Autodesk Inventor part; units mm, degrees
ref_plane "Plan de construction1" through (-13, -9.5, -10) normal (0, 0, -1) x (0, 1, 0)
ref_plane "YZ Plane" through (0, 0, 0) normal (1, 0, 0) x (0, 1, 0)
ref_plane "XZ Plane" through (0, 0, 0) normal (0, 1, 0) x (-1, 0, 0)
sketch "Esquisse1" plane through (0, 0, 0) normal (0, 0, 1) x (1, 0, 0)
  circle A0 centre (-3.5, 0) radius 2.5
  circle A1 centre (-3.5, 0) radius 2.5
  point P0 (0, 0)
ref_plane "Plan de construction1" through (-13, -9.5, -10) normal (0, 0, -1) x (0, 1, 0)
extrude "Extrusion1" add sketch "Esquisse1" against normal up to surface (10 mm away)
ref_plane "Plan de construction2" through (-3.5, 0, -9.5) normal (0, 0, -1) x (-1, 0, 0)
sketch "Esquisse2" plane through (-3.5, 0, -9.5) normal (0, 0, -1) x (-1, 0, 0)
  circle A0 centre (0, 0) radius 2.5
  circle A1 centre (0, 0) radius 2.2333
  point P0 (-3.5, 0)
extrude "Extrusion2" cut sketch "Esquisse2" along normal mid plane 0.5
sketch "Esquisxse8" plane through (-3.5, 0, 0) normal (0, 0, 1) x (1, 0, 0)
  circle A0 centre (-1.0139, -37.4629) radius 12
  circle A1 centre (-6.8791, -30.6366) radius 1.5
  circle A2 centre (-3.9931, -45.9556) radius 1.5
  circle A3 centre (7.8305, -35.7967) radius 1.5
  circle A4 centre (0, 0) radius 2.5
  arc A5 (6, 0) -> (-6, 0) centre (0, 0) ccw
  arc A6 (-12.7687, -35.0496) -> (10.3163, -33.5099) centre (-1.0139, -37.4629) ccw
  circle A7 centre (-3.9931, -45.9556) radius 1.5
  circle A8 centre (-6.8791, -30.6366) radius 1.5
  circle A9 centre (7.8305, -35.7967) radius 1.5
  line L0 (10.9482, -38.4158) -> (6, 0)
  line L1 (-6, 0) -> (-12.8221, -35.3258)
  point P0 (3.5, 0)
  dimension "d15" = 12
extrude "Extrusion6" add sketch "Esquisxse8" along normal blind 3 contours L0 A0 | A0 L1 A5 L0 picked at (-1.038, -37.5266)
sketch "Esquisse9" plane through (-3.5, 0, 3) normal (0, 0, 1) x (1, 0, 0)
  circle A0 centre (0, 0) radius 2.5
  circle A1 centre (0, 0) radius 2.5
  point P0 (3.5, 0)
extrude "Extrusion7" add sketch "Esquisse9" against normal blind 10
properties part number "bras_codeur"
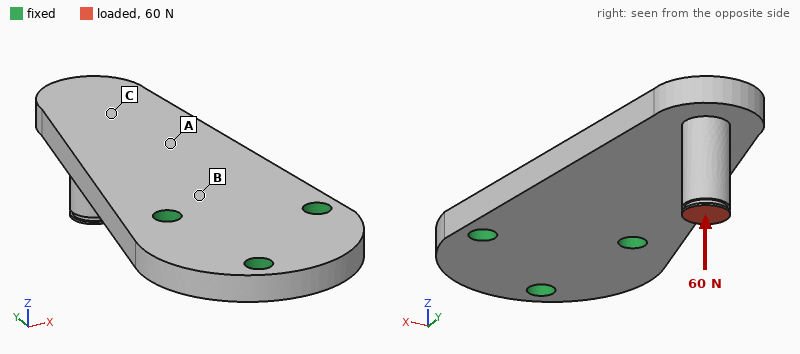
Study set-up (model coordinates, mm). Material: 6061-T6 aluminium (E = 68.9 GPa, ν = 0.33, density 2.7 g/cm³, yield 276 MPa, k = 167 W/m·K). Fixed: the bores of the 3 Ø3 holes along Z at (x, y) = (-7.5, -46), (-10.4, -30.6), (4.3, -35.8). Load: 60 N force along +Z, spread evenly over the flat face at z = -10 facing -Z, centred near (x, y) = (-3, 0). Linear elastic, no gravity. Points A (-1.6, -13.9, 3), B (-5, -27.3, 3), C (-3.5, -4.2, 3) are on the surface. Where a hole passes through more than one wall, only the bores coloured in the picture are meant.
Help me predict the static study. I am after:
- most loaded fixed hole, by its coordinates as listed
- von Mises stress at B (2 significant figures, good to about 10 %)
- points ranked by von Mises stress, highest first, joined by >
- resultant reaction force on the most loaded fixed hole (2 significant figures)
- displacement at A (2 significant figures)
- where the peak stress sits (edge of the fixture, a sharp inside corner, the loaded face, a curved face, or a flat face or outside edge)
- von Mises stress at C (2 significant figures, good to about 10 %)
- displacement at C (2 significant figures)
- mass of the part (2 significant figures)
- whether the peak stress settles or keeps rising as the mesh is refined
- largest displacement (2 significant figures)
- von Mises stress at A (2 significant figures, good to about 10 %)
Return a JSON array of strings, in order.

["(-10.4, -30.6)", "47 MPa", "B > A > C", "89 N", "0.084 mm", "edge of the fixture", "14 MPa", "0.17 mm", "8.1 g", "keeps rising", "0.28 mm", "33 MPa"]
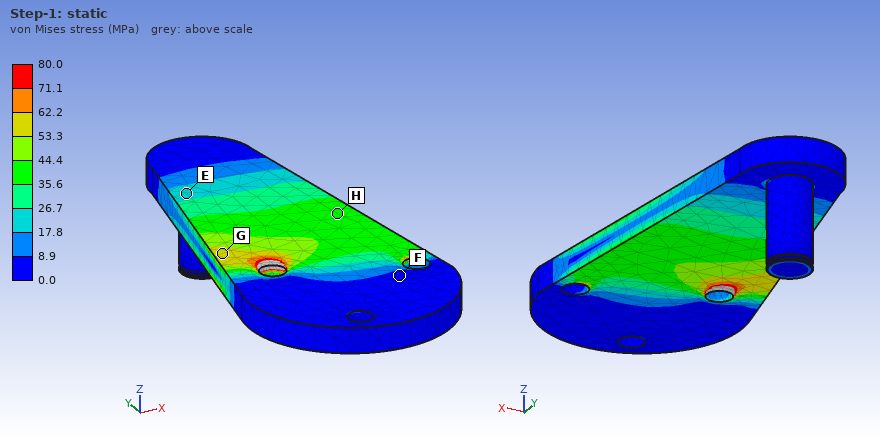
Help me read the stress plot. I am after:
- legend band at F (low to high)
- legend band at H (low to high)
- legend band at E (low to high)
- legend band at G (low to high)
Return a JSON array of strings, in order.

["0.0 to 8.9 MPa", "35.6 to 44.4 MPa", "17.8 to 26.7 MPa", "53.3 to 62.2 MPa"]
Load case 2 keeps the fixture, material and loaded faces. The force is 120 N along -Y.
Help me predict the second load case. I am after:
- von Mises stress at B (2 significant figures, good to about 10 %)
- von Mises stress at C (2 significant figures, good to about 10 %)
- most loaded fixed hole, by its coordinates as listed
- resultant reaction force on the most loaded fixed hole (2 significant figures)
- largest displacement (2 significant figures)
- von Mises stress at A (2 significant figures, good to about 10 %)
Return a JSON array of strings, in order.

["39 MPa", "65 MPa", "(-10.4, -30.6)", "69 N", "0.36 mm", "52 MPa"]
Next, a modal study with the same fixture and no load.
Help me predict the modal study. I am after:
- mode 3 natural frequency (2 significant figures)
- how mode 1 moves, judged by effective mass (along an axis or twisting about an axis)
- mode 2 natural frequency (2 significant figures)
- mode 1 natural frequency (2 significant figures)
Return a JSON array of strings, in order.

["9300 Hz", "along Z", "7300 Hz", "1900 Hz"]
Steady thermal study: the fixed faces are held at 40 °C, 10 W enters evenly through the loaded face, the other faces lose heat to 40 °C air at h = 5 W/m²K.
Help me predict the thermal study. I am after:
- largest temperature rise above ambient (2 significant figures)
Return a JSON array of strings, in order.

["73 K"]
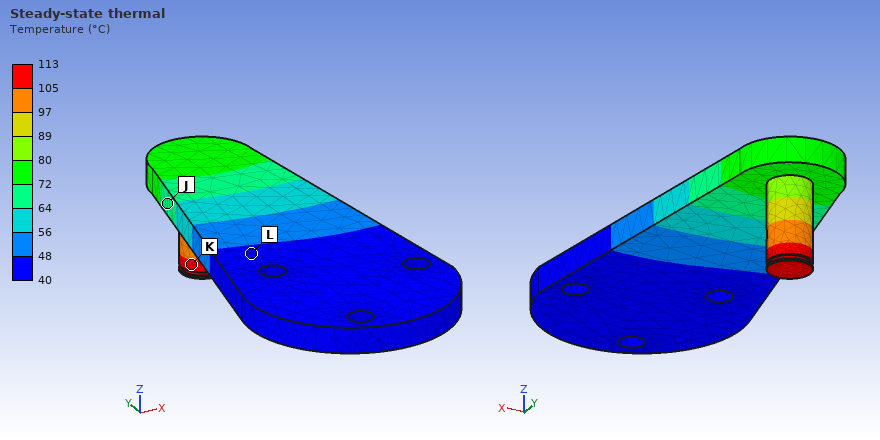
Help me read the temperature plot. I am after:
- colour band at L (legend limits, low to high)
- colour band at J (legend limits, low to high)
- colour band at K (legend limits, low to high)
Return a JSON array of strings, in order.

["40 to 48 °C", "64 to 72 °C", "105 to 113 °C"]
